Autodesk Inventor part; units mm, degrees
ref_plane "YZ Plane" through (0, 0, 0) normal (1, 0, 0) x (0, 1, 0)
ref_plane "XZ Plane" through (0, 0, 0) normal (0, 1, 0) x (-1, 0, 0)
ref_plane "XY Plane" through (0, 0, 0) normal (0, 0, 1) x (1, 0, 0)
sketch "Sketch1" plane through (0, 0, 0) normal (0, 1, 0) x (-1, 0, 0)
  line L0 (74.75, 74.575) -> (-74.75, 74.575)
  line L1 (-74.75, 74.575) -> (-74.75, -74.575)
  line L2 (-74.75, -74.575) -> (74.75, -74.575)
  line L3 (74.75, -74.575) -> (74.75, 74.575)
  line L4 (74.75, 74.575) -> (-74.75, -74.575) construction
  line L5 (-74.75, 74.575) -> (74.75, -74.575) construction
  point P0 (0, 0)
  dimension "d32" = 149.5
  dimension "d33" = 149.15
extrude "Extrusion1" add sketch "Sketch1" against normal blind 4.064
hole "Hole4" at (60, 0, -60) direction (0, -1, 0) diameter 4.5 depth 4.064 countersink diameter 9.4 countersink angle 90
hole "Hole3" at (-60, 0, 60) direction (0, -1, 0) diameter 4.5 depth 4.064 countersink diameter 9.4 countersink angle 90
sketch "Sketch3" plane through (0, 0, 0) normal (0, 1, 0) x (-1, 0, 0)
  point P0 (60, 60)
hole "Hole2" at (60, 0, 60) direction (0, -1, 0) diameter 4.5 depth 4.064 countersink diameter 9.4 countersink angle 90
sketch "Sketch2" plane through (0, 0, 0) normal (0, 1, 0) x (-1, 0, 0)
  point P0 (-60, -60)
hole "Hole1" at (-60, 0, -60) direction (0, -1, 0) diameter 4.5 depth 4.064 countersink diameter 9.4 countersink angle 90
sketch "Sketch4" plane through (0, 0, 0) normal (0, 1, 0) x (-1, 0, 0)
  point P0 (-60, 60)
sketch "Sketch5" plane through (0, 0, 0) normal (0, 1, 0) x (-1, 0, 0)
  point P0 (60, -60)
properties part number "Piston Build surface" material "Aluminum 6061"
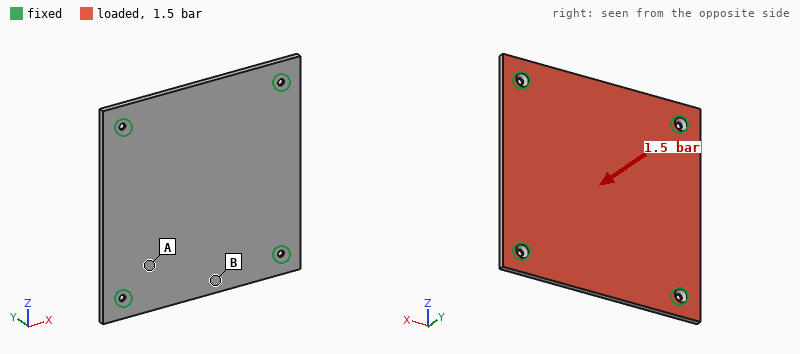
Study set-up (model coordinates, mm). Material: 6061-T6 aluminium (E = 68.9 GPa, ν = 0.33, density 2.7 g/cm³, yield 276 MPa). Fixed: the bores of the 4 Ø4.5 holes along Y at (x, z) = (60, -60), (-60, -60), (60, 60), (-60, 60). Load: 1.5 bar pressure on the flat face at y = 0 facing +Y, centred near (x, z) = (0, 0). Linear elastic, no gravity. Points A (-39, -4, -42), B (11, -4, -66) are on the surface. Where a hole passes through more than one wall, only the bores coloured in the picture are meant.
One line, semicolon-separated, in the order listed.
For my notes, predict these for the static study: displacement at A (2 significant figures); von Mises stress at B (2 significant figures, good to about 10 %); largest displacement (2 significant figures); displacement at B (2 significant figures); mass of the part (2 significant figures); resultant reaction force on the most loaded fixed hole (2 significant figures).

0.34 mm; 46 MPa; 0.75 mm; 0.38 mm; 240 g; 2.0 kN
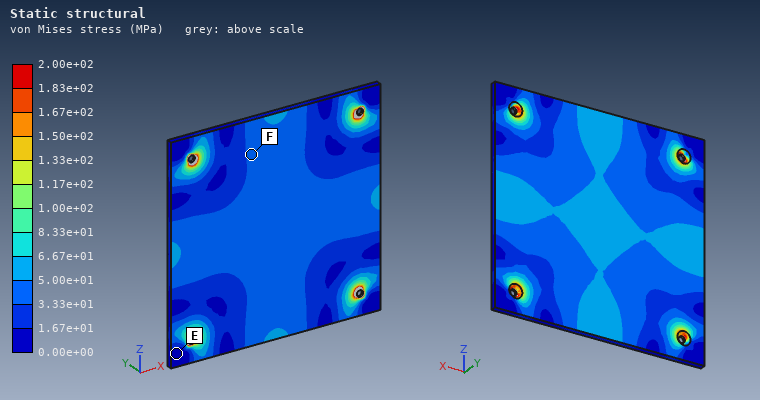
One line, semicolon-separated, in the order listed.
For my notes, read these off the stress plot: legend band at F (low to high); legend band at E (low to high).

3.33e+01 to 5.00e+01 MPa; 0.00e+00 to 1.67e+01 MPa
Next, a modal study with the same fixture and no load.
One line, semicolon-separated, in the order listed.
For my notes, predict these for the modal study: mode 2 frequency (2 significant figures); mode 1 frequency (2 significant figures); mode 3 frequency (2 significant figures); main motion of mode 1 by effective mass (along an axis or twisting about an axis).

1400 Hz; 820 Hz; 1400 Hz; along Y
